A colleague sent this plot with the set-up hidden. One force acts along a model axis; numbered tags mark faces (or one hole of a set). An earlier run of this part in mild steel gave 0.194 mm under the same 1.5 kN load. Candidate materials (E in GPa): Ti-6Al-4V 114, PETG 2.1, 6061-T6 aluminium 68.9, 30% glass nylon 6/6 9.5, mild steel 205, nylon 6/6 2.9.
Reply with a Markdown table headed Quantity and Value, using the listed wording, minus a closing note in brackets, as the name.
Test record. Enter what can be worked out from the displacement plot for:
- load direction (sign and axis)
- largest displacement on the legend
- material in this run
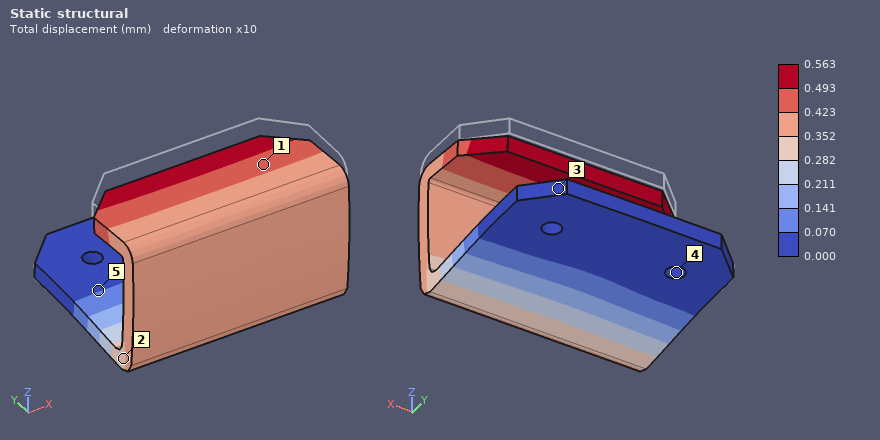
| Quantity | Value |
|---|---|
| load direction | -Z |
| largest displacement on the legend | 0.563 mm |
| material in this run | 6061-T6 aluminium |
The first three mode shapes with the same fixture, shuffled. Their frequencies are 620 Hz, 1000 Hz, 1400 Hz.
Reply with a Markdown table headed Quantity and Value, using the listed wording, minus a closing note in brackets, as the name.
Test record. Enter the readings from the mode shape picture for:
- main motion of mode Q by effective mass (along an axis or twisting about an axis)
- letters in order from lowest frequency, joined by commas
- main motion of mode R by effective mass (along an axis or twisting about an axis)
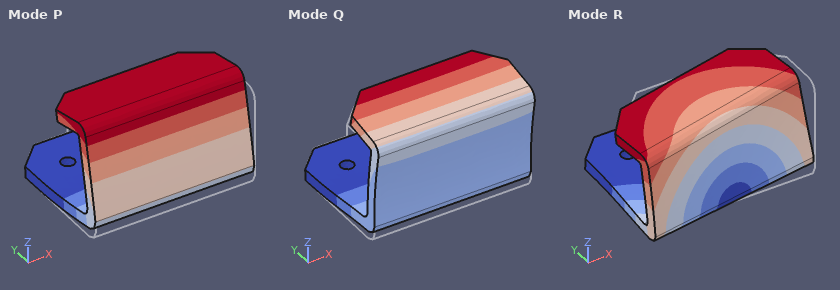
| Quantity | Value |
|---|---|
| main motion of mode Q by effective mass | along Z |
| letters in order from lowest frequency, joined by commas | P, R, Q |
| main motion of mode R by effective mass | along X |
